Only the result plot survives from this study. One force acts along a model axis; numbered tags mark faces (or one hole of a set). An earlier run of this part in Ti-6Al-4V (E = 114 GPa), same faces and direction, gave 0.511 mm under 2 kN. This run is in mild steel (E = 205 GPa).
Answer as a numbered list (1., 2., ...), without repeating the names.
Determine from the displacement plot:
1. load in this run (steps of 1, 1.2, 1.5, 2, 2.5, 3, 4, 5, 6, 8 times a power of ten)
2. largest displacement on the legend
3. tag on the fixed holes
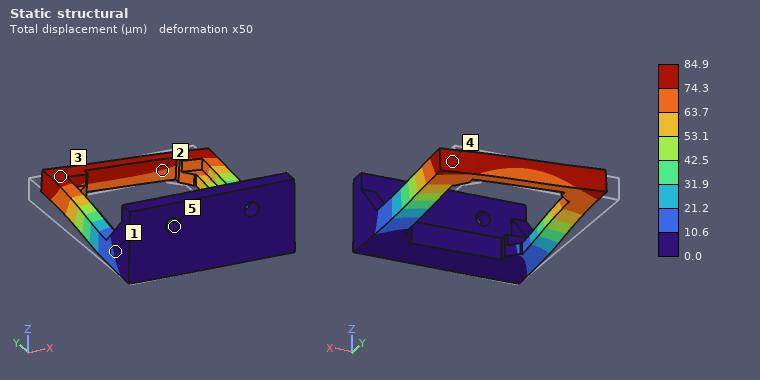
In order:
1. 600 N
2. 84.9 µm
3. 5
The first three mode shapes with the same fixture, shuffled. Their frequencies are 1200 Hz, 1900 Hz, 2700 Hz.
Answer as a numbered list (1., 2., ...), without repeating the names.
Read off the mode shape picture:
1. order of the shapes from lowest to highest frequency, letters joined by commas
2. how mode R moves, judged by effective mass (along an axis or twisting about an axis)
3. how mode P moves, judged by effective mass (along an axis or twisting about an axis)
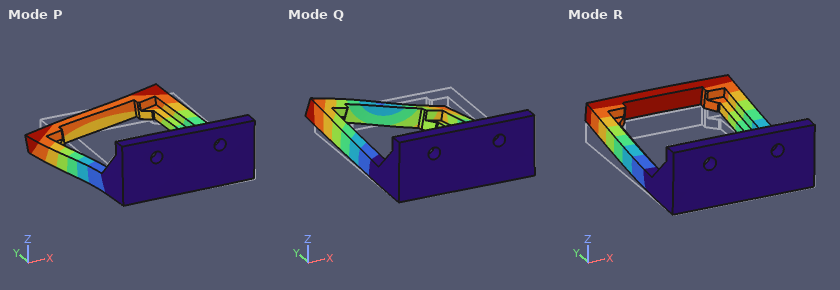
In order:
1. R, P, Q
2. along Z
3. along X
